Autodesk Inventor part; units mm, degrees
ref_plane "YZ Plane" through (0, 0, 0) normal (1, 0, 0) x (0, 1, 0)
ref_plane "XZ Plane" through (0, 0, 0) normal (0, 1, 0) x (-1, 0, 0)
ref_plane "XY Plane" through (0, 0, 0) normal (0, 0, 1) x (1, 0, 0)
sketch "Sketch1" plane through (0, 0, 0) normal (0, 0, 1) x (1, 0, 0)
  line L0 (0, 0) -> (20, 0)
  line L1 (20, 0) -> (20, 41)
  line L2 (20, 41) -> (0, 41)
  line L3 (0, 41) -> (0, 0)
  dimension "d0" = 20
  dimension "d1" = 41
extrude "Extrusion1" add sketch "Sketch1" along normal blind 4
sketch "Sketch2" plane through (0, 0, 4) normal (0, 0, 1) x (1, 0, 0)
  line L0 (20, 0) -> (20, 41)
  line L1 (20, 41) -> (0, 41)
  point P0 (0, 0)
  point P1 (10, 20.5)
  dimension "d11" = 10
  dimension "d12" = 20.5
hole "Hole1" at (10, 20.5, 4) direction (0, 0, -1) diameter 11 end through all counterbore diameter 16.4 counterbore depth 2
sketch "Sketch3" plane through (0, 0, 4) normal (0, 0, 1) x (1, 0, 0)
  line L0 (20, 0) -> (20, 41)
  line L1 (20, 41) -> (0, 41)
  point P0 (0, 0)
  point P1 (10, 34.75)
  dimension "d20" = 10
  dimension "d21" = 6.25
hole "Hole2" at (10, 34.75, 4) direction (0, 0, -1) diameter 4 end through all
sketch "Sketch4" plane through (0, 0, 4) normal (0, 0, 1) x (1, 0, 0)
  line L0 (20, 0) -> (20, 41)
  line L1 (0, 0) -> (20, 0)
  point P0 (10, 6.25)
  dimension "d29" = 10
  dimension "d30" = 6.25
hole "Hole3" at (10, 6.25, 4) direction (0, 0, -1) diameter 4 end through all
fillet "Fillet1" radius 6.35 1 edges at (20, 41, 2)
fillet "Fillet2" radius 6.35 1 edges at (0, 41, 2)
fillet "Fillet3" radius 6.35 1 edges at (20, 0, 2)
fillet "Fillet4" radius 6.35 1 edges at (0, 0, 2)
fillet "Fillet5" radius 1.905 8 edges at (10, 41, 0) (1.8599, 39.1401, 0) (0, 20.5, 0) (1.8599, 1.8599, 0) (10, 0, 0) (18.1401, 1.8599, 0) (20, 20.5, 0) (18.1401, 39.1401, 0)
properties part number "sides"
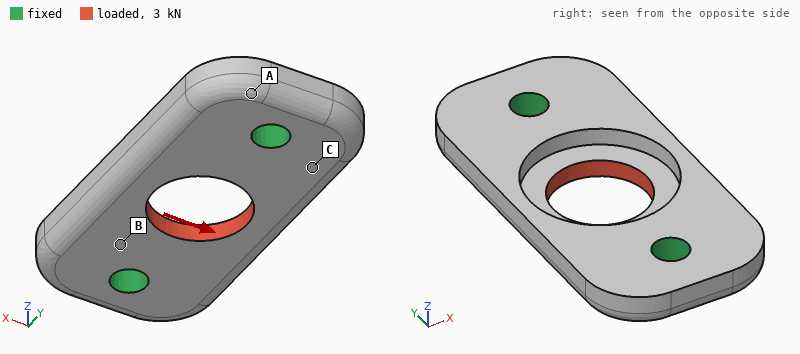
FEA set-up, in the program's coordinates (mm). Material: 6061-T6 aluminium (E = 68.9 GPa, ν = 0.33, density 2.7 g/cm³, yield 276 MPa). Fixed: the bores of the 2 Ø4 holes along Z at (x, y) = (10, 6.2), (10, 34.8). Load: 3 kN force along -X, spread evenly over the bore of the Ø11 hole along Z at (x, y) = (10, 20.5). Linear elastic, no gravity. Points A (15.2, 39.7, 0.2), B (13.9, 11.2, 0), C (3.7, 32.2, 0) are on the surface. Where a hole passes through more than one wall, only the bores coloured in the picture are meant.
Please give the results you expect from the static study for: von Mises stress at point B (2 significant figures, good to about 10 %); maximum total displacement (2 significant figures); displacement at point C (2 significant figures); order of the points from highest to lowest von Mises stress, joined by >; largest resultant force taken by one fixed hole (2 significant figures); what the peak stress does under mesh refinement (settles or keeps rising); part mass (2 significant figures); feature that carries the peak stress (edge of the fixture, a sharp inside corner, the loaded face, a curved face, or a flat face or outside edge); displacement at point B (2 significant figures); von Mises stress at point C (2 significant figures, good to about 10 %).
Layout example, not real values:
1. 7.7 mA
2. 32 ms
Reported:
1. 58 MPa
2. 25 µm
3. 6.7 µm
4. B > C > A
5. 1.5 kN
6. keeps rising
7. 6.3 g
8. edge of the fixture
9. 8.5 µm
10. 32 MPa
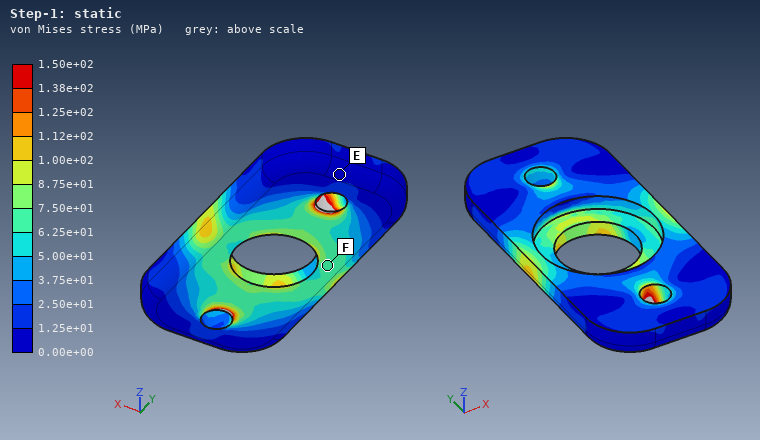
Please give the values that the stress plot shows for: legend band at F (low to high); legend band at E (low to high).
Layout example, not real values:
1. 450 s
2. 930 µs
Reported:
1. 6.25e+01 to 7.50e+01 MPa
2. 0.00e+00 to 1.25e+01 MPa
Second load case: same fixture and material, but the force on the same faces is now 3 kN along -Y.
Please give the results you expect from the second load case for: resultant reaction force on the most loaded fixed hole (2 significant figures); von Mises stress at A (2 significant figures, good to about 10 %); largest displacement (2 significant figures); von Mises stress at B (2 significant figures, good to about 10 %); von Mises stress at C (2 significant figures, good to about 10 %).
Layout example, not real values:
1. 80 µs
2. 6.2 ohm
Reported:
1. 1.5 kN
2. 6.5 MPa
3. 9.7 µm
4. 44 MPa
5. 21 MPa
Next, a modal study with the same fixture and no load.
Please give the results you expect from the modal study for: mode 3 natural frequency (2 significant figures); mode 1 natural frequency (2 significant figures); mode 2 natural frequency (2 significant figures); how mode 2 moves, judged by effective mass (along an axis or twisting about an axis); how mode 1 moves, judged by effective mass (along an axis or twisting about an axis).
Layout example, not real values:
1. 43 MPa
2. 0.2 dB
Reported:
1. 34 kHz
2. 21 kHz
3. 23 kHz
4. along Z
5. twisting about Y
